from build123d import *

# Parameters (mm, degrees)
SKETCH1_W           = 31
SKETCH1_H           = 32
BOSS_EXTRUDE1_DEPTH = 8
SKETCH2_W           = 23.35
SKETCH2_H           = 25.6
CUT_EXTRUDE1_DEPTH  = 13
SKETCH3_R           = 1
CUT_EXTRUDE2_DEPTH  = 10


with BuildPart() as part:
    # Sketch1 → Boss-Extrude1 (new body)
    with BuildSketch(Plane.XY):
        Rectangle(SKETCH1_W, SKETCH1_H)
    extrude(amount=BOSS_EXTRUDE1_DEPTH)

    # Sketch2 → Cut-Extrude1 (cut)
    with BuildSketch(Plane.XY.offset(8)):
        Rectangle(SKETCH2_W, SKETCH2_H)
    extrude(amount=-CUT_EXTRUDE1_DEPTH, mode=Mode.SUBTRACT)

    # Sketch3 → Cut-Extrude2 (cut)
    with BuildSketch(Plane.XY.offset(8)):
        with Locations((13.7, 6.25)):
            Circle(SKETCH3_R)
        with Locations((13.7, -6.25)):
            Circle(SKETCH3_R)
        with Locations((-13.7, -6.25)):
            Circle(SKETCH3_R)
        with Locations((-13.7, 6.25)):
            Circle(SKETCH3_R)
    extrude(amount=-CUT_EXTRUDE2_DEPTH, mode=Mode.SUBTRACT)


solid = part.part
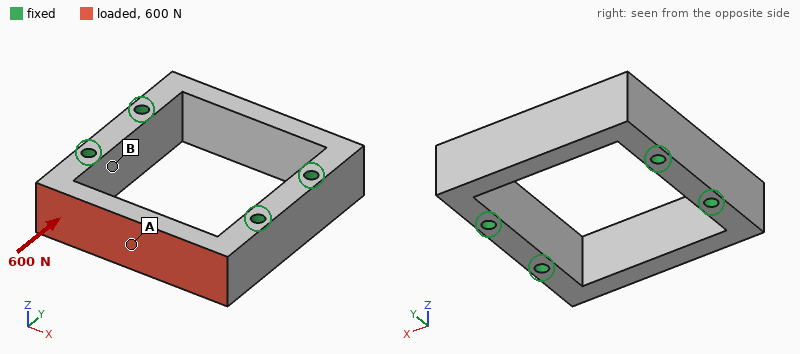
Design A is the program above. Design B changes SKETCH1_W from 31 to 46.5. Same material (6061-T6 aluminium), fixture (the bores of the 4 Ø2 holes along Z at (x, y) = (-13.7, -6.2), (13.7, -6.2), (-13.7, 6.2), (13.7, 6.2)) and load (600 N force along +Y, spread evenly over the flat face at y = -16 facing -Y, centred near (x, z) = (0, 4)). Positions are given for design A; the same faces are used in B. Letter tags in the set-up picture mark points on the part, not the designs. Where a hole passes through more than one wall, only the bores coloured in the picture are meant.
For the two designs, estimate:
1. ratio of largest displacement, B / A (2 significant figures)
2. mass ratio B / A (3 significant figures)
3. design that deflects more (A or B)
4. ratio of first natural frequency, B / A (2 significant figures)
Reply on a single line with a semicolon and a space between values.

0.58; 2.30; A; 1.1
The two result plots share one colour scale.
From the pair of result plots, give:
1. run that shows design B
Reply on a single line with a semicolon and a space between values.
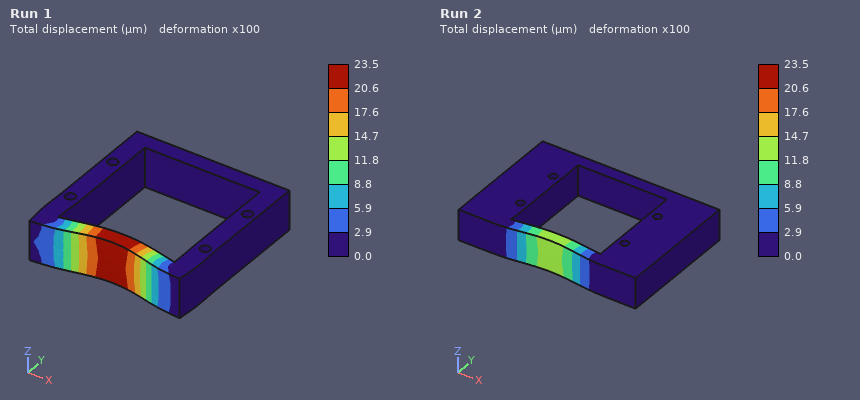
Run 2
